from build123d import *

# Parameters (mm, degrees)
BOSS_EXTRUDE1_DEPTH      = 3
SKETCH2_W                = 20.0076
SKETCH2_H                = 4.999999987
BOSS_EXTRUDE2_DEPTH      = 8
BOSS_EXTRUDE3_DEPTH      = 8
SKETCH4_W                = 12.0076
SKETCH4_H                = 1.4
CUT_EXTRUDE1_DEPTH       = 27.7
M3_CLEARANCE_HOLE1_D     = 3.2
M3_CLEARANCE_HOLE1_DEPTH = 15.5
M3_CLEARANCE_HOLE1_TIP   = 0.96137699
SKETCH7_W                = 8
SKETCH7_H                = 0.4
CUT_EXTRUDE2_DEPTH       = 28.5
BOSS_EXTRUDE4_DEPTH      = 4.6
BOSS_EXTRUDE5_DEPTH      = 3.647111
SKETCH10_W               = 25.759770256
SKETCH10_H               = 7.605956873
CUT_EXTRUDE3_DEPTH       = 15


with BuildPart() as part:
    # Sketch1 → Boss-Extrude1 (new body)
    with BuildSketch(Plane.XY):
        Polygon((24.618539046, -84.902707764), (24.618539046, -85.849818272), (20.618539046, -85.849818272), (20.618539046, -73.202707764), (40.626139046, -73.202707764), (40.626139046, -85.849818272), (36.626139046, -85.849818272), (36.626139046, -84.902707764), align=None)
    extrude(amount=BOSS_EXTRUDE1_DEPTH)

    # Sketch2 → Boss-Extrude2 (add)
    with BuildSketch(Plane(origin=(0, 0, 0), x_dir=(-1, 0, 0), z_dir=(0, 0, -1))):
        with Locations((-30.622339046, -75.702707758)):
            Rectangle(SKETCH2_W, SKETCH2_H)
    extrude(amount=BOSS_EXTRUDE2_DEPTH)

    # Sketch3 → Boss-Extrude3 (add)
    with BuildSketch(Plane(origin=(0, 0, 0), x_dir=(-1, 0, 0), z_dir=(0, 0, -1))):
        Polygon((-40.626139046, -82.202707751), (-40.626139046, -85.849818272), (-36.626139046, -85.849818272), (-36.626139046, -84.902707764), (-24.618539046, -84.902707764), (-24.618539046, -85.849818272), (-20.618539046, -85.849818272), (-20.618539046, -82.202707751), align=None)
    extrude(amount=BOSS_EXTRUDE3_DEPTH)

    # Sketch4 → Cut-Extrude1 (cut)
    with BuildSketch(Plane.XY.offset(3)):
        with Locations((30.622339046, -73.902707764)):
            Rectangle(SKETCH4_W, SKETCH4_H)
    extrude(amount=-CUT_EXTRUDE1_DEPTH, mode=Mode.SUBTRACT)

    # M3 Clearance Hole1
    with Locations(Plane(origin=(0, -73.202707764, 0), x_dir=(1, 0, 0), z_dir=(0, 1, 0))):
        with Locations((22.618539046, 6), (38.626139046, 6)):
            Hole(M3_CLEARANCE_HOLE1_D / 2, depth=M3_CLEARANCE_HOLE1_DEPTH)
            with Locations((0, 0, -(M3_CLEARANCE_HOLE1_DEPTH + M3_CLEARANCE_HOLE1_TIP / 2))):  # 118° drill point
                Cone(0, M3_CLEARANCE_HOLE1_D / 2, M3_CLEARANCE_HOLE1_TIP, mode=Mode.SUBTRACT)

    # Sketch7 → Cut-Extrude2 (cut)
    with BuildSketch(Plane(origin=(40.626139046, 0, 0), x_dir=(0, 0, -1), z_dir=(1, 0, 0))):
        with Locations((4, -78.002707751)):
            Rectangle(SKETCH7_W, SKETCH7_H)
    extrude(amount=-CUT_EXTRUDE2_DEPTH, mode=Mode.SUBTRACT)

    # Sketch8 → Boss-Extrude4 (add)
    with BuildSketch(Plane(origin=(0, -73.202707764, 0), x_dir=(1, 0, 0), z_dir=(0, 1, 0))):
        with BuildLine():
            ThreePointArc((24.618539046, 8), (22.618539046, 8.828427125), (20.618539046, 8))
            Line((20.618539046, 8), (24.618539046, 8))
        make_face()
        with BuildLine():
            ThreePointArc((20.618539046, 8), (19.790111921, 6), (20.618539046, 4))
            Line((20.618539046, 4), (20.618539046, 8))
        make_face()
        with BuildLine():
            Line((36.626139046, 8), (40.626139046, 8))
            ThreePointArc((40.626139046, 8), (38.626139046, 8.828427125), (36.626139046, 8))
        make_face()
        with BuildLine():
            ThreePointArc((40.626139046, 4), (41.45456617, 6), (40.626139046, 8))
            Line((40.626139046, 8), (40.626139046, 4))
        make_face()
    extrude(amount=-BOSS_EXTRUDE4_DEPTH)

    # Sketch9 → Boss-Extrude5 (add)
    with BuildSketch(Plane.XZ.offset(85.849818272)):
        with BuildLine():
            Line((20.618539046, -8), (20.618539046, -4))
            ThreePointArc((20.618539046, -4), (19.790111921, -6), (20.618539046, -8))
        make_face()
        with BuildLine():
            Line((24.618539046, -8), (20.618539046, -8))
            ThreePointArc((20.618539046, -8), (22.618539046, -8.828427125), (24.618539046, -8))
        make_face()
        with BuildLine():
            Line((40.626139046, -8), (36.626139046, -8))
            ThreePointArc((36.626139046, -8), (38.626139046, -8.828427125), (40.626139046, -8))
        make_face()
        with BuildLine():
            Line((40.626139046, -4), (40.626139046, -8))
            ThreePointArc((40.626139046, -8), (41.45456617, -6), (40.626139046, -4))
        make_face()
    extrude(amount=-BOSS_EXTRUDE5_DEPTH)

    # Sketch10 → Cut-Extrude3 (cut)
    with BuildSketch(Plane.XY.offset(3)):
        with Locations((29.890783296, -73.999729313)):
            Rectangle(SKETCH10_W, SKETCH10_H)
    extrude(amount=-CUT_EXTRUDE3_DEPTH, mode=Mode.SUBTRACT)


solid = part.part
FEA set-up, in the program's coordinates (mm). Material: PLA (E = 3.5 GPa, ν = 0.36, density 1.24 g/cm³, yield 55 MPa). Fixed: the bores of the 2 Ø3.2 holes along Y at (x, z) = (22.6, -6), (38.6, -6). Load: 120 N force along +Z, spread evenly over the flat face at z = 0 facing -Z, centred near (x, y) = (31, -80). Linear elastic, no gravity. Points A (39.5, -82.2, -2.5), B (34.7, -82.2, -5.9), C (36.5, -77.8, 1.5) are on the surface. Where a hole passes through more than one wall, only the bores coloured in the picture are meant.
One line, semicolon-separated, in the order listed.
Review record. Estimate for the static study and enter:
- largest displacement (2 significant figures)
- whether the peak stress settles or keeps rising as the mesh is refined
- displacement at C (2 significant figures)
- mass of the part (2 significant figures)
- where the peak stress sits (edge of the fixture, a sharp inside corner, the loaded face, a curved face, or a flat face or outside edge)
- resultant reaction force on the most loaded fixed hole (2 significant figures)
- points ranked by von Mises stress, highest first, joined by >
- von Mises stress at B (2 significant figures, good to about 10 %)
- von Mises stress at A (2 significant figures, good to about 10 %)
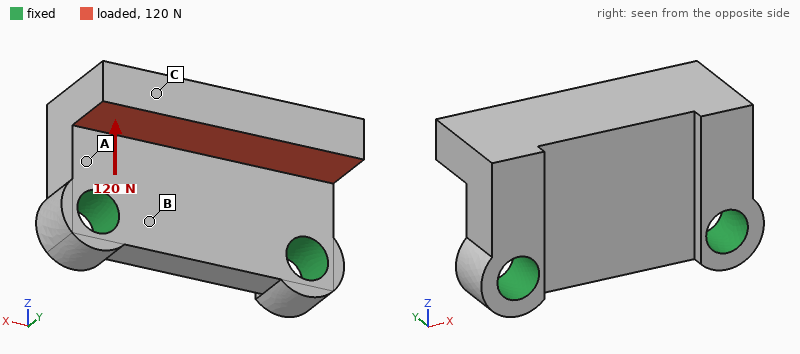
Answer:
0.15 mm; keeps rising; 0.13 mm; 1.1 g; edge of the fixture; 64 N; A > B > C; 7.3 MPa; 18 MPa
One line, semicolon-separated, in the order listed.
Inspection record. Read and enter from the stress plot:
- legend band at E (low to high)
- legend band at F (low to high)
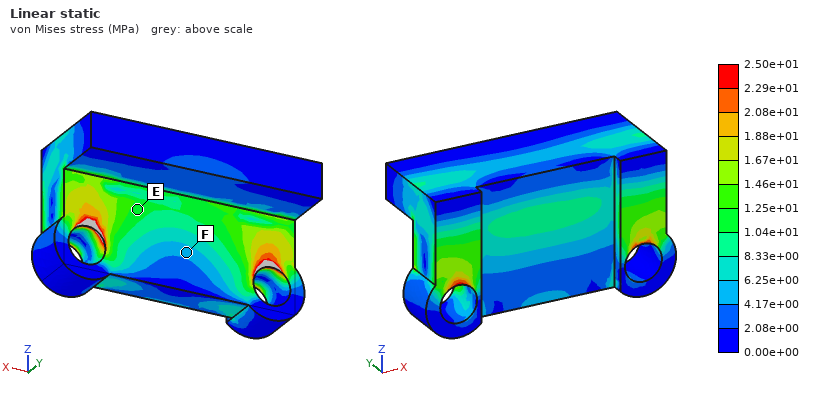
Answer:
1.04e+01 to 1.25e+01 MPa; 4.17e+00 to 6.25e+00 MPa
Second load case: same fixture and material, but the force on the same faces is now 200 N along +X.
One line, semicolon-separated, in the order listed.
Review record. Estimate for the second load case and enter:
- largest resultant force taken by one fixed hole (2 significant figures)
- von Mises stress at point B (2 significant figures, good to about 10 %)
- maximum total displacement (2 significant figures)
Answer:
130 N; 4.9 MPa; 100 µm
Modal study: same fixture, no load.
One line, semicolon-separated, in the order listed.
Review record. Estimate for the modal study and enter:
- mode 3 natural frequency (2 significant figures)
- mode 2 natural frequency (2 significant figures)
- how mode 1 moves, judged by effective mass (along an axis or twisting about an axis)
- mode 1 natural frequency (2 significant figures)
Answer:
17 kHz; 11 kHz; along Y; 6500 Hz
